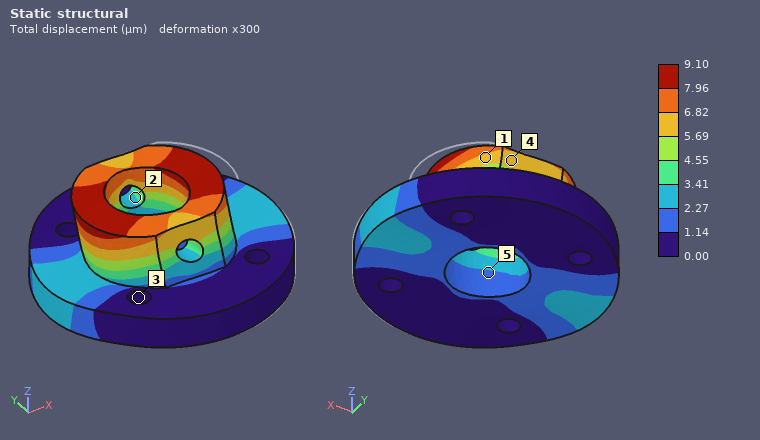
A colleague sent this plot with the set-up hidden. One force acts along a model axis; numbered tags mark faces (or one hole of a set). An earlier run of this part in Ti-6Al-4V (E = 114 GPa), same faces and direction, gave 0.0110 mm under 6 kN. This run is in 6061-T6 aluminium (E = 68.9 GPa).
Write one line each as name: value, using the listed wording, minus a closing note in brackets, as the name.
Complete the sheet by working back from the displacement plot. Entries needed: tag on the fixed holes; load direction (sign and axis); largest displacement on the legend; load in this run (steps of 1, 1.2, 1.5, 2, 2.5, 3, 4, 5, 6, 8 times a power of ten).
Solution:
tag on the fixed holes: 3
load direction: -X
largest displacement on the legend: 9.10 µm
load in this run: 3 kN
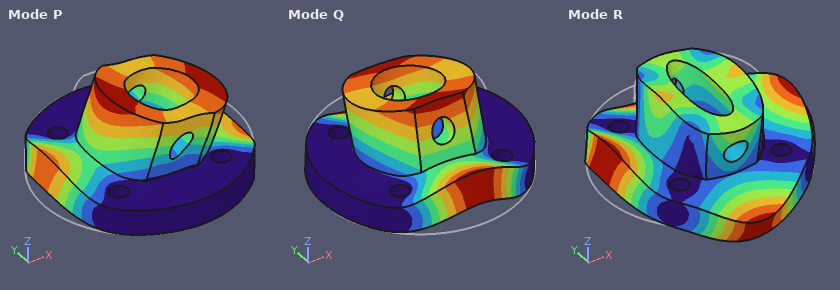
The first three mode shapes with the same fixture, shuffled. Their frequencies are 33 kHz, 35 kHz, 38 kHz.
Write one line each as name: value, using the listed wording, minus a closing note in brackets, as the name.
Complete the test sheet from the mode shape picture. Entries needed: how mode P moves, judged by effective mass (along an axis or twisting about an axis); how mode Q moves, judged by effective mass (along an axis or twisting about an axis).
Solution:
how mode P moves, judged by effective mass: along X
how mode Q moves, judged by effective mass: along Y
